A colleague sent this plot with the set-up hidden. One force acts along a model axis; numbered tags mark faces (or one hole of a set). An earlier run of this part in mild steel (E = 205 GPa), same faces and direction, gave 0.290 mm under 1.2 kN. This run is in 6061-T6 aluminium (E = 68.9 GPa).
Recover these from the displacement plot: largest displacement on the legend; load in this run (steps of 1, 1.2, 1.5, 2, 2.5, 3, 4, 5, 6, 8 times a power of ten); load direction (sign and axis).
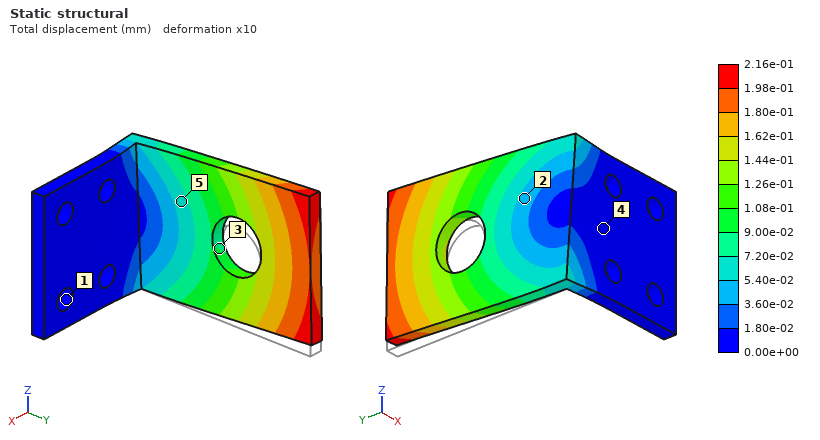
2.16e-01 mm
300 N
+Z
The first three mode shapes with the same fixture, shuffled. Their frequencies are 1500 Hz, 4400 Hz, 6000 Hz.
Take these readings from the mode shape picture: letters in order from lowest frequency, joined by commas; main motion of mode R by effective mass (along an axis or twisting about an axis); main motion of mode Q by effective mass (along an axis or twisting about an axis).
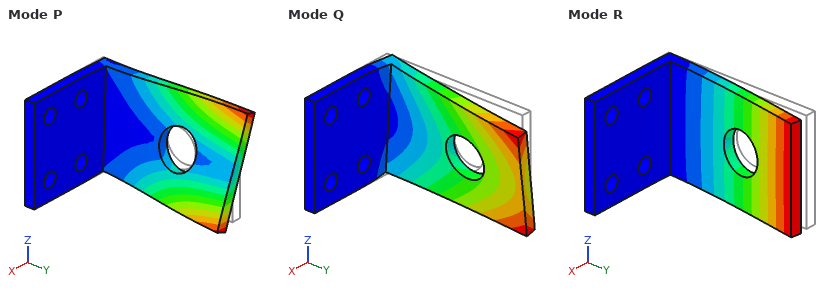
R, Q, P
along X
along Z
